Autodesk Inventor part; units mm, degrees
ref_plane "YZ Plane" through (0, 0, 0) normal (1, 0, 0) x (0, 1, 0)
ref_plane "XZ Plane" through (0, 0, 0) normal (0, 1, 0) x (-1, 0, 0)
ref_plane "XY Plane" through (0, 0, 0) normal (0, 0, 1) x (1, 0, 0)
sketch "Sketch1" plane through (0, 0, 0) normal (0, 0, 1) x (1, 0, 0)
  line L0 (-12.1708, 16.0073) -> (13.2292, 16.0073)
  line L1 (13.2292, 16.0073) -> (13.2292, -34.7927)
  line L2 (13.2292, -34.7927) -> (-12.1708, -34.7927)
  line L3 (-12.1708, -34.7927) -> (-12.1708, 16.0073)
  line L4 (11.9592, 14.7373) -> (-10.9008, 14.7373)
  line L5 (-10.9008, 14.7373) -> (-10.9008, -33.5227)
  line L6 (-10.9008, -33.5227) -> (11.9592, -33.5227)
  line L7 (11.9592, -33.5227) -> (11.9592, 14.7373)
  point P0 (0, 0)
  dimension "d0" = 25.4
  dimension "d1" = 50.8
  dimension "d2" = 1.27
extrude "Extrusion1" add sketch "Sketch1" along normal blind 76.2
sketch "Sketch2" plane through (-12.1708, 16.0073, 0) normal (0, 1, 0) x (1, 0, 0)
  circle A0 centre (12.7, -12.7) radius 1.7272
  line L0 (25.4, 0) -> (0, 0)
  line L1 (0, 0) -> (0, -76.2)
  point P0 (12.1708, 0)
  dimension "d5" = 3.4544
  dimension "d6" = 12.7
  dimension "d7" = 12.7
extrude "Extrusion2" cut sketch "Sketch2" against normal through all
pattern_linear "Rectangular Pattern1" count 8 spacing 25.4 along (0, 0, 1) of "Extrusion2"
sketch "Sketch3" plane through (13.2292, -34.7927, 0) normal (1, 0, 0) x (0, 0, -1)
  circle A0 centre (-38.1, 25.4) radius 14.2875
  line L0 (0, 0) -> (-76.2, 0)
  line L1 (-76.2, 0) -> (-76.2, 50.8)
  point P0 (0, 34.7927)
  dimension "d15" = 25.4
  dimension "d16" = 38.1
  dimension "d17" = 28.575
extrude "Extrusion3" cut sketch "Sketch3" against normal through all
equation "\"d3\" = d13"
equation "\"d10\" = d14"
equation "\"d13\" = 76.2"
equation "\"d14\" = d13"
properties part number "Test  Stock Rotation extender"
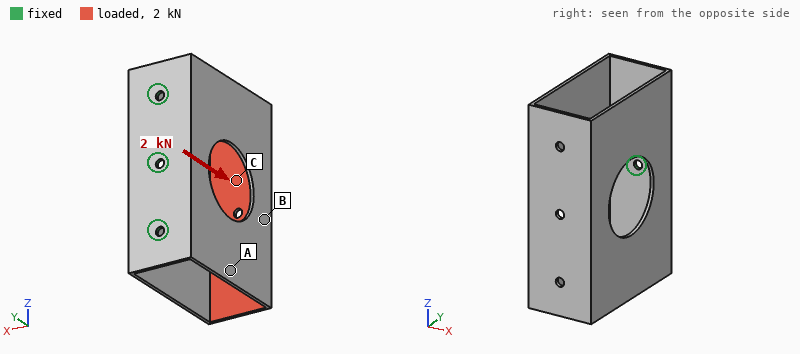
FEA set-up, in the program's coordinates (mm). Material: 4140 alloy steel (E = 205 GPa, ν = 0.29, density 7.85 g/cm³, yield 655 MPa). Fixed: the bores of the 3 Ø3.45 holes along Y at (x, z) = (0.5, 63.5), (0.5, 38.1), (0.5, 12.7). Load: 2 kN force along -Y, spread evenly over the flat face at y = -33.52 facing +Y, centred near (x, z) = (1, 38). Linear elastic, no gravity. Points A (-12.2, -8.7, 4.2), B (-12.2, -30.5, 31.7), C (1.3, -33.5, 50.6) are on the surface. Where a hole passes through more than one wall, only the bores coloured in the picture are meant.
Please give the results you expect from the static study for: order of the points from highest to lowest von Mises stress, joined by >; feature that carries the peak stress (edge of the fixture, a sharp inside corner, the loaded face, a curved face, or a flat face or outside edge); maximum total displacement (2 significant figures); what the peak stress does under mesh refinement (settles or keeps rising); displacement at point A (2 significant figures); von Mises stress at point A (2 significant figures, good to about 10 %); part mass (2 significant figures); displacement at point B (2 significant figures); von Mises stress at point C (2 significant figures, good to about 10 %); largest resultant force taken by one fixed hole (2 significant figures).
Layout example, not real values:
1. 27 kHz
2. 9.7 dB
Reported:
1. C > A > B
2. edge of the fixture
3. 0.28 mm
4. keeps rising
5. 0.26 mm
6. 88 MPa
7. 99 g
8. 0.16 mm
9. 250 MPa
10. 690 N
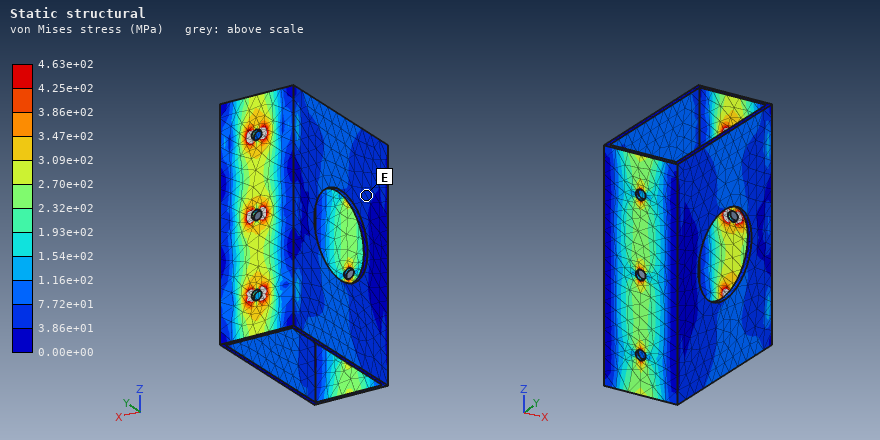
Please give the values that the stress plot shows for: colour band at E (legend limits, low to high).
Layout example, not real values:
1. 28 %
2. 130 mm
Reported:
1. 3.86e+01 to 7.72e+01 MPa
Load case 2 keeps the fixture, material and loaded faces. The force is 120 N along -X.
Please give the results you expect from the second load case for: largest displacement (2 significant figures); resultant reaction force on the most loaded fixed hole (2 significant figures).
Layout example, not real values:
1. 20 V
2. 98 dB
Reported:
1. 0.73 mm
2. 50 N
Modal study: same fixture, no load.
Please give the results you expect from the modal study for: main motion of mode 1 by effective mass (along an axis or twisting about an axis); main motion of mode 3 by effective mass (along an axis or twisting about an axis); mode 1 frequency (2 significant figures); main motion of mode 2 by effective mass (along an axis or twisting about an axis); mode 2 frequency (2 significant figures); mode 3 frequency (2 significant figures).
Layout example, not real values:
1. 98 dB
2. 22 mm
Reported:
1. along X
2. along Z
3. 320 Hz
4. twisting about Y
5. 1100 Hz
6. 1100 Hz
